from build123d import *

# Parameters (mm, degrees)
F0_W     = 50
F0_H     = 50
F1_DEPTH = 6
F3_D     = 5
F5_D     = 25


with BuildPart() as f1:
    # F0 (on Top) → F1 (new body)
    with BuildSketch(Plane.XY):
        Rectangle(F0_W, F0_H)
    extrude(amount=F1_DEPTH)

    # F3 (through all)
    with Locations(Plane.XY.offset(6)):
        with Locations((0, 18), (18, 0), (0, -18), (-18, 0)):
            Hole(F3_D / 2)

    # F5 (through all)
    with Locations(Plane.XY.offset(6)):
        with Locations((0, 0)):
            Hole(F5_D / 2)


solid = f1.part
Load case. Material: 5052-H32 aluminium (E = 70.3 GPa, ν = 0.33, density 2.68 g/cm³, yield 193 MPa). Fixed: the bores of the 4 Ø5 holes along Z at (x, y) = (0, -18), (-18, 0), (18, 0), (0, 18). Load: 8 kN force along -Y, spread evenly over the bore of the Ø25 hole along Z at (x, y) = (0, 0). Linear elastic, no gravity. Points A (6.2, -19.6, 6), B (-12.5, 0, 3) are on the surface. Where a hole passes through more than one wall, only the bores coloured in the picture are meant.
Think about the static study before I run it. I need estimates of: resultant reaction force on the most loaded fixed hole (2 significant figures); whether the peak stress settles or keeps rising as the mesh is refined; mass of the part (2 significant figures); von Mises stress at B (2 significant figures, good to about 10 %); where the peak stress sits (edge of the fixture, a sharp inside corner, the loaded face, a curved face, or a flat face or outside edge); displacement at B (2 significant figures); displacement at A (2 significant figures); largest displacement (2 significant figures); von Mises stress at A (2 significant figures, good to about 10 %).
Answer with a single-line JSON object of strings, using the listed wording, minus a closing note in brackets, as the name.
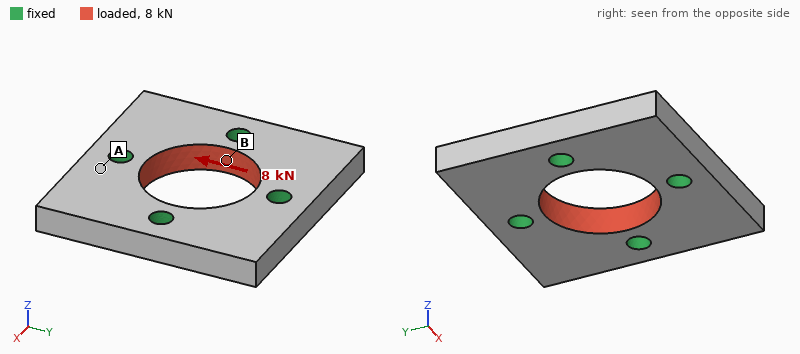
{"resultant reaction force on the most loaded fixed hole": "2.1 kN", "whether the peak stress settles or keeps rising as the mesh is refined": "keeps rising", "mass of the part": "31 g", "von Mises stress at B": "29 MPa", "where the peak stress sits": "edge of the fixture", "displacement at B": "3.1 µm", "displacement at A": "1.6 µm", "largest displacement": "4.1 µm", "von Mises stress at A": "14 MPa"}
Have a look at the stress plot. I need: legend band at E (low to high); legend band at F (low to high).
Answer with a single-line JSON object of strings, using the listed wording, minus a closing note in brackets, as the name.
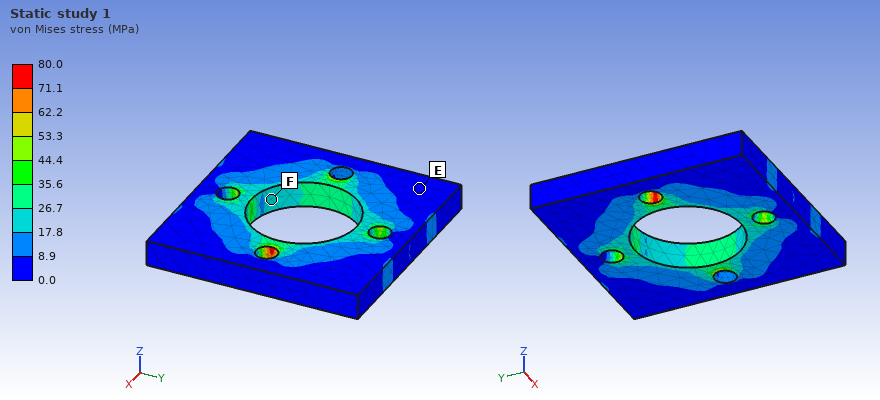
{"legend band at E": "0.0 to 8.9 MPa", "legend band at F": "17.8 to 26.7 MPa"}
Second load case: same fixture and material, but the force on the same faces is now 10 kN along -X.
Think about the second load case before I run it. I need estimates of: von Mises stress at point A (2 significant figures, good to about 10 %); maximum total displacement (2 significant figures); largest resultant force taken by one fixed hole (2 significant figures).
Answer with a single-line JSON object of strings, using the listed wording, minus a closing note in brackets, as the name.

{"von Mises stress at point A": "14 MPa", "maximum total displacement": "5.1 µm", "largest resultant force taken by one fixed hole": "2.7 kN"}
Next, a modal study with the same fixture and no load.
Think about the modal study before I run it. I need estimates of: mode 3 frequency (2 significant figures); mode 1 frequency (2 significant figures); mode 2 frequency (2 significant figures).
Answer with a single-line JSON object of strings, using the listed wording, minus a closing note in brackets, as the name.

{"mode 3 frequency": "14 kHz", "mode 1 frequency": "14 kHz", "mode 2 frequency": "14 kHz"}
